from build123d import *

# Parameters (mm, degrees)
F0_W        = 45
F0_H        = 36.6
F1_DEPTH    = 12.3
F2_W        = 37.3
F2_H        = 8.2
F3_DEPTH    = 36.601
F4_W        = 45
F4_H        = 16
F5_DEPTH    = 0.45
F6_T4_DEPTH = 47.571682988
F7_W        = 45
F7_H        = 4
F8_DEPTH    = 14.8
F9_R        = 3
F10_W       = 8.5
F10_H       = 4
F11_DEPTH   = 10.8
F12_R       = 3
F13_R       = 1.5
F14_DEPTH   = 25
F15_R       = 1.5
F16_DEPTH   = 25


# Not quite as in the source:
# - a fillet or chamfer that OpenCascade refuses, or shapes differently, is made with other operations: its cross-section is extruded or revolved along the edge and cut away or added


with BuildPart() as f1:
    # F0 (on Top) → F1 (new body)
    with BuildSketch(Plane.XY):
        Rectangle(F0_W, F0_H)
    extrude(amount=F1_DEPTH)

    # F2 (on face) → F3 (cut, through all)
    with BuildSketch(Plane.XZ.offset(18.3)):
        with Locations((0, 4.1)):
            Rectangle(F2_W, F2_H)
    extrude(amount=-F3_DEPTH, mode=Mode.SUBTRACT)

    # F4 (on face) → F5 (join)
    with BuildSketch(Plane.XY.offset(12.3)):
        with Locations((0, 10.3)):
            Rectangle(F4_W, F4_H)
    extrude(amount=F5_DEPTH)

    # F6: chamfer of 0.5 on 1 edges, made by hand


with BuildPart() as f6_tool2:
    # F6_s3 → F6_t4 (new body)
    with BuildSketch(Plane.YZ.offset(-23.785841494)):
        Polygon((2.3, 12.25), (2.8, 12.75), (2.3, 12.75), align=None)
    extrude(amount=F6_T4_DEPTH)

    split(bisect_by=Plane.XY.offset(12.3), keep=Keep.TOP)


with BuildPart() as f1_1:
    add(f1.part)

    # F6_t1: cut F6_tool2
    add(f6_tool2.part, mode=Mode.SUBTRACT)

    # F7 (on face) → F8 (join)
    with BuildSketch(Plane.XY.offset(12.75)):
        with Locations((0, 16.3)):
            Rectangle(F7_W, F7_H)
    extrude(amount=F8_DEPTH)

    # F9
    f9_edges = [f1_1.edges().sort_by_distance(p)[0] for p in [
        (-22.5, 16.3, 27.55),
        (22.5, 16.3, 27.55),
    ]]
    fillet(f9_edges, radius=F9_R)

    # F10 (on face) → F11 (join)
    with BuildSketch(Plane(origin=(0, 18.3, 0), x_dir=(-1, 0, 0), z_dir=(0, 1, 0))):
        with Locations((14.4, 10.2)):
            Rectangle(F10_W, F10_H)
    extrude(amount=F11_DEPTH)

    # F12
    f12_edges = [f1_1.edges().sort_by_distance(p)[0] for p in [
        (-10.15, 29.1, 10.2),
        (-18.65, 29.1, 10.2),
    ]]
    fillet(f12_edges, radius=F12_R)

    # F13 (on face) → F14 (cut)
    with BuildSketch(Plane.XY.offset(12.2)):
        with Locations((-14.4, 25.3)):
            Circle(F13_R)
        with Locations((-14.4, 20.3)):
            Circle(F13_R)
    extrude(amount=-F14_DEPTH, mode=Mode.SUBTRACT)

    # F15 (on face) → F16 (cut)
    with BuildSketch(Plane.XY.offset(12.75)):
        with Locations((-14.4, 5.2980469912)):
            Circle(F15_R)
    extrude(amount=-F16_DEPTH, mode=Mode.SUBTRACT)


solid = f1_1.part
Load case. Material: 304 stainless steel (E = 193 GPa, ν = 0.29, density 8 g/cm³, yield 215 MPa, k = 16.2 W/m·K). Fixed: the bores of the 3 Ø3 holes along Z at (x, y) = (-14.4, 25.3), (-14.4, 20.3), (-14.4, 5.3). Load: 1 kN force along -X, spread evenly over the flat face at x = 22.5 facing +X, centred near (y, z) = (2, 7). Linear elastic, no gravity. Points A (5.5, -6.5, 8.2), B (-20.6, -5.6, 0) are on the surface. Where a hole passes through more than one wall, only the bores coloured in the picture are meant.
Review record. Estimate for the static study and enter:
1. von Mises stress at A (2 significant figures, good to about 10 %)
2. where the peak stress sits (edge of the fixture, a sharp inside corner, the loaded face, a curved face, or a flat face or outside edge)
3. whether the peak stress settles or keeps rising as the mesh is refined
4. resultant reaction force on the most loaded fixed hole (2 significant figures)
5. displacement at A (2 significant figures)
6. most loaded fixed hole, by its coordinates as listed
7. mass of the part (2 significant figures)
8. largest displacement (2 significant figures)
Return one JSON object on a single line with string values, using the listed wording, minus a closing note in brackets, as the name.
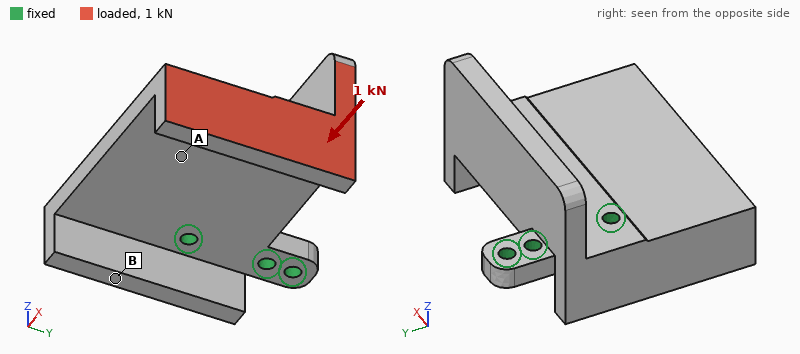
{"von Mises stress at A": "21 MPa", "where the peak stress sits": "edge of the fixture", "whether the peak stress settles or keeps rising as the mesh is refined": "keeps rising", "resultant reaction force on the most loaded fixed hole": "1.2 kN", "displacement at A": "9.0 µm", "most loaded fixed hole, by its coordinates as listed": "(-14.4, 5.3)", "mass of the part": "98 g", "largest displacement": "37 µm"}
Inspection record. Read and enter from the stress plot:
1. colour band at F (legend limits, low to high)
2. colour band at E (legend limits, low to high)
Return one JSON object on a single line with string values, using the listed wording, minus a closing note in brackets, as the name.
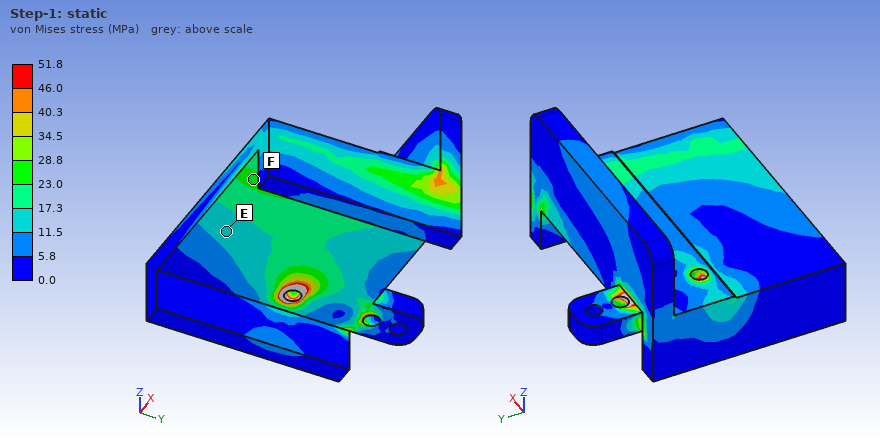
{"colour band at F": "23.0 to 28.8 MPa", "colour band at E": "11.5 to 17.3 MPa"}
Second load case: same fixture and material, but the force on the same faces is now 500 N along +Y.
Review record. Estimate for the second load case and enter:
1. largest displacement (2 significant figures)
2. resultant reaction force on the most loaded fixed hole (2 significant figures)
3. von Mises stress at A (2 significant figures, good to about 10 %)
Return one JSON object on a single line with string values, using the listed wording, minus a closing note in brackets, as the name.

{"largest displacement": "28 µm", "resultant reaction force on the most loaded fixed hole": "1.1 kN", "von Mises stress at A": "11 MPa"}
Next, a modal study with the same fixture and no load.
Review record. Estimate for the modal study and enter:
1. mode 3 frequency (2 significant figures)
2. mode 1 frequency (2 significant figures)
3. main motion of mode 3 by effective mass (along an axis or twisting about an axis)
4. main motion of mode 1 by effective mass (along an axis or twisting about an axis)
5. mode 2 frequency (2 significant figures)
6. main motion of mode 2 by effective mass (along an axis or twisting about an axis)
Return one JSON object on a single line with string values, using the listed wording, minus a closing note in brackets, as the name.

{"mode 3 frequency": "5100 Hz", "mode 1 frequency": "2100 Hz", "main motion of mode 3 by effective mass": "along Y", "main motion of mode 1 by effective mass": "along Z", "mode 2 frequency": "3900 Hz", "main motion of mode 2 by effective mass": "twisting about X"}
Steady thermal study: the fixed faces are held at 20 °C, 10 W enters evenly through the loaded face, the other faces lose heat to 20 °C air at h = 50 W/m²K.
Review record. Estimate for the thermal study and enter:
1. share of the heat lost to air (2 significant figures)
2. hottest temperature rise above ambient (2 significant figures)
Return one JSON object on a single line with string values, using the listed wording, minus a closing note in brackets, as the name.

{"share of the heat lost to air": "73 %", "hottest temperature rise above ambient": "71 K"}
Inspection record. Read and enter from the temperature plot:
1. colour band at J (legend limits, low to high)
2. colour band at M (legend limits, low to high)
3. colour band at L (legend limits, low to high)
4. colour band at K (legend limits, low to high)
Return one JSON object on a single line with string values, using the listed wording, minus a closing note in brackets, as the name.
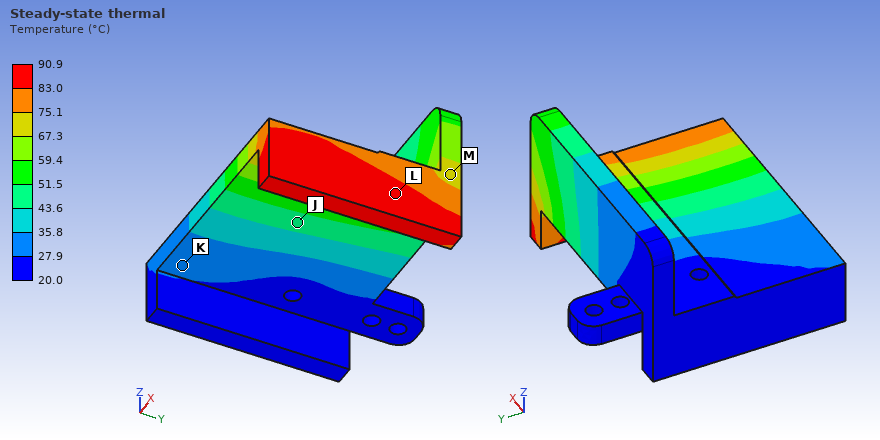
{"colour band at J": "43.6 to 51.5 °C", "colour band at M": "67.3 to 75.1 °C", "colour band at L": "83.0 to 90.9 °C", "colour band at K": "27.9 to 35.8 °C"}
